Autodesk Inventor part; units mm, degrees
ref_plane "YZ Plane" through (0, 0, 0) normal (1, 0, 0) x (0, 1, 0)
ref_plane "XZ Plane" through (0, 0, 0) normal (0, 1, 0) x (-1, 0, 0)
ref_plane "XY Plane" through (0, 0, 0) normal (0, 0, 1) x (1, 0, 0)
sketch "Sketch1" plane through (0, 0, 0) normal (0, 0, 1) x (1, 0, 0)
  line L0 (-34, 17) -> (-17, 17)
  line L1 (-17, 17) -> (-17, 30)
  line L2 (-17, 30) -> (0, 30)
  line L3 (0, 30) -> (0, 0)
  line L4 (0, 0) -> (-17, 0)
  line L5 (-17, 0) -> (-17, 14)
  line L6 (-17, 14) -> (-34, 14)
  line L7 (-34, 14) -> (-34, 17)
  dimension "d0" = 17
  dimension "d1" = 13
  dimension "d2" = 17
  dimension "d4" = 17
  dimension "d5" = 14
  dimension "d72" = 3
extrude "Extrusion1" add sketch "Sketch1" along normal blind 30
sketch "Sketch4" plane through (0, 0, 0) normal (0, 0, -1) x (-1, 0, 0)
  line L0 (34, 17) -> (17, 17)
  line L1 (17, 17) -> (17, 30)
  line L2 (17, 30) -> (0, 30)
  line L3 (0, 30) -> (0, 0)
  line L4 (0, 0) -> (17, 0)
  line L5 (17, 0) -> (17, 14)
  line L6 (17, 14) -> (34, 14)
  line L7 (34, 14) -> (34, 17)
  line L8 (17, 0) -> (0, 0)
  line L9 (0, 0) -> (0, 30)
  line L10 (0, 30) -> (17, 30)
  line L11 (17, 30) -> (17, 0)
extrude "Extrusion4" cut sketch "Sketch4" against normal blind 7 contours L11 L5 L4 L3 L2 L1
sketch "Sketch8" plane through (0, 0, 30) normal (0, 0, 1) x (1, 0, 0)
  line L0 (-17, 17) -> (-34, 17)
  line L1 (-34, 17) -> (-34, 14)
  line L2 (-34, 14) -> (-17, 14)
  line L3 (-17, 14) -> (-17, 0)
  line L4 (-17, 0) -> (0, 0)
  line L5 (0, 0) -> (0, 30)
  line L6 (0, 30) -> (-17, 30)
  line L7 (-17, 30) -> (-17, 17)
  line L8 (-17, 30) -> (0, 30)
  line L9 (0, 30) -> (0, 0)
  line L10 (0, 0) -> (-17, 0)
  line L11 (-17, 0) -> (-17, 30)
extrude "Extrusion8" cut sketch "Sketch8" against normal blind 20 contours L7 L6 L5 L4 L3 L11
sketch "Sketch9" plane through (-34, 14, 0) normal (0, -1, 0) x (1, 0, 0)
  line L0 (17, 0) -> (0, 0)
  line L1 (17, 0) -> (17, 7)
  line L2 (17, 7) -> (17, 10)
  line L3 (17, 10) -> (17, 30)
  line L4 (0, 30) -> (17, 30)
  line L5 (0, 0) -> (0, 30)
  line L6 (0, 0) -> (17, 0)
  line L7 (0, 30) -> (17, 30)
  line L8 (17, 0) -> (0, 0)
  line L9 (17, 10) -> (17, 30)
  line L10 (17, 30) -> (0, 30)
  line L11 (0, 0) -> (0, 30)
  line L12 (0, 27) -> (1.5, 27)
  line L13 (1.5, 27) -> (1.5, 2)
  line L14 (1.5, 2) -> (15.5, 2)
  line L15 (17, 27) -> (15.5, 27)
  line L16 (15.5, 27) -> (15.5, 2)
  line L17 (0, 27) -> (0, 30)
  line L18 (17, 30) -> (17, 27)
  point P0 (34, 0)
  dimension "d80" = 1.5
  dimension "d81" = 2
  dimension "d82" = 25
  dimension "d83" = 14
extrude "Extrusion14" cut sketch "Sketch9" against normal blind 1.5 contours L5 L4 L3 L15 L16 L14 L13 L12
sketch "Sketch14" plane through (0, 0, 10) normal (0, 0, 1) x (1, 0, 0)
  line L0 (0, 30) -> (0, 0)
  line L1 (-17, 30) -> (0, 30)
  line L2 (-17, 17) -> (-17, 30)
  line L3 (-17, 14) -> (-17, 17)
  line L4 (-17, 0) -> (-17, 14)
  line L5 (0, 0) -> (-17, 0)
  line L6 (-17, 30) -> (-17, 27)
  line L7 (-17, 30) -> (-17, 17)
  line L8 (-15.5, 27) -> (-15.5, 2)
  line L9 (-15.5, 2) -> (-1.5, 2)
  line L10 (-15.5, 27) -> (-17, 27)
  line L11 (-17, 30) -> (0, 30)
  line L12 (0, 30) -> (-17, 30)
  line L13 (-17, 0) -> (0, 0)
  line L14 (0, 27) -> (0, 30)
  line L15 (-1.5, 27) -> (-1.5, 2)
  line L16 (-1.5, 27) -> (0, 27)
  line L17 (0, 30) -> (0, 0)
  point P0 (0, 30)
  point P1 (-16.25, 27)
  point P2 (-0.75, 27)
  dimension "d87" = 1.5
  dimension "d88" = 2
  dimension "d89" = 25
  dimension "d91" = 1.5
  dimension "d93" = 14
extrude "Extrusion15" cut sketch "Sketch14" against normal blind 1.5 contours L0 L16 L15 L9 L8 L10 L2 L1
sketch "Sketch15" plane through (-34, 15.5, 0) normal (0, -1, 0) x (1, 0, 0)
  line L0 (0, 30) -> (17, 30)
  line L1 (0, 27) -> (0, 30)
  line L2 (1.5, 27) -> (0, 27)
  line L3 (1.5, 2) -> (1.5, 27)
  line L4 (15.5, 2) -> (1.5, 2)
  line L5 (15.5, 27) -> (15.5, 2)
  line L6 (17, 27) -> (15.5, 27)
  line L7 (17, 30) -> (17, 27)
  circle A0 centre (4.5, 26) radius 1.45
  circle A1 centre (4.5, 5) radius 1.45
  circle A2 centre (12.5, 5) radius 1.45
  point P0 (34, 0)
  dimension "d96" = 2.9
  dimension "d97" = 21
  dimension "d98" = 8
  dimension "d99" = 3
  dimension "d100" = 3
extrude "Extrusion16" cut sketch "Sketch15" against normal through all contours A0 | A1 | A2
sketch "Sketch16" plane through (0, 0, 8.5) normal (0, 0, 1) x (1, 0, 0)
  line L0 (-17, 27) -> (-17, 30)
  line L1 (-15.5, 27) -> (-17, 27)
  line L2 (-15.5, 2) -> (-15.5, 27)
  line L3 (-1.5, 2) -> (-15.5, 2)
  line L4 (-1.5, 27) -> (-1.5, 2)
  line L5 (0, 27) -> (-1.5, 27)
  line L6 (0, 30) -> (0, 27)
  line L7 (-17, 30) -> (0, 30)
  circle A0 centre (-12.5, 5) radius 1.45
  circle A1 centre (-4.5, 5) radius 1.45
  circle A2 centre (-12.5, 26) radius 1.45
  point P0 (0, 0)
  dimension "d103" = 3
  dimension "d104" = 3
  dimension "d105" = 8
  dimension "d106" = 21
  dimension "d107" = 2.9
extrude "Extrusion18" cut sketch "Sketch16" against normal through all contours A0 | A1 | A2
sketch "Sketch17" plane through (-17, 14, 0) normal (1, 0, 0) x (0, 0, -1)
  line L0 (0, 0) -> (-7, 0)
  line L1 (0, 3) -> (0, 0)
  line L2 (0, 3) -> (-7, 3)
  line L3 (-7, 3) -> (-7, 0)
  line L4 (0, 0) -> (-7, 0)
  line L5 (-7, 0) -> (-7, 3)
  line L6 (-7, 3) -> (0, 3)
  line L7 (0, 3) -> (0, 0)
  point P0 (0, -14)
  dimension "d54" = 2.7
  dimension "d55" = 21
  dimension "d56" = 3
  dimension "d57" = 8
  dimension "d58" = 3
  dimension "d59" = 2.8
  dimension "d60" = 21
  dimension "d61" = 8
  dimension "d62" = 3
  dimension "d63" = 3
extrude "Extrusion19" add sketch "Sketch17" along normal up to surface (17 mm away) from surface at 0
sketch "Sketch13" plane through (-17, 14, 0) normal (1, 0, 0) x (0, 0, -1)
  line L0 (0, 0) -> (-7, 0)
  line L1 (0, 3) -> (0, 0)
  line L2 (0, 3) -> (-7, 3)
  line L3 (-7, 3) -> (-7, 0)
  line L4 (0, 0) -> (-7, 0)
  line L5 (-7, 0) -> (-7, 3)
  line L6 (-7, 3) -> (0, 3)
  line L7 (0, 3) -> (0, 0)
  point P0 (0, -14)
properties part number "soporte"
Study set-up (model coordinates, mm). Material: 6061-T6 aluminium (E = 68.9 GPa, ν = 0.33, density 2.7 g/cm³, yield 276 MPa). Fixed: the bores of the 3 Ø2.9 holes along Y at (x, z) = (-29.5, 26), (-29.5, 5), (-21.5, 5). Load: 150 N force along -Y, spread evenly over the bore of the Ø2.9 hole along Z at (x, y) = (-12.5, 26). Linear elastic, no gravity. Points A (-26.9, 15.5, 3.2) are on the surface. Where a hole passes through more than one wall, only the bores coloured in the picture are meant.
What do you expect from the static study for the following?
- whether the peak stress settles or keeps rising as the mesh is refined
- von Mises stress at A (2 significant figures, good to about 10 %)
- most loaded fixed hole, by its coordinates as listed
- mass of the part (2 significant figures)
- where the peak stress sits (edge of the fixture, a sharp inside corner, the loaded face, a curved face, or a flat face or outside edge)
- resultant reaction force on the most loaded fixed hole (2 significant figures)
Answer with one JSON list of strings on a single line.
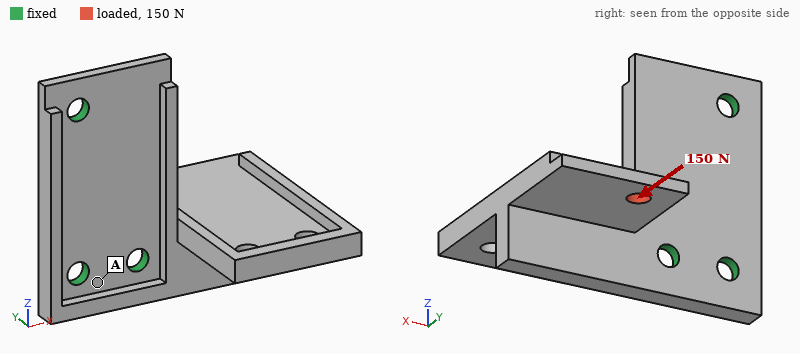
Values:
["keeps rising", "17 MPa", "(-21.5, 5)", "5.8 g", "edge of the fixture", "220 N"]
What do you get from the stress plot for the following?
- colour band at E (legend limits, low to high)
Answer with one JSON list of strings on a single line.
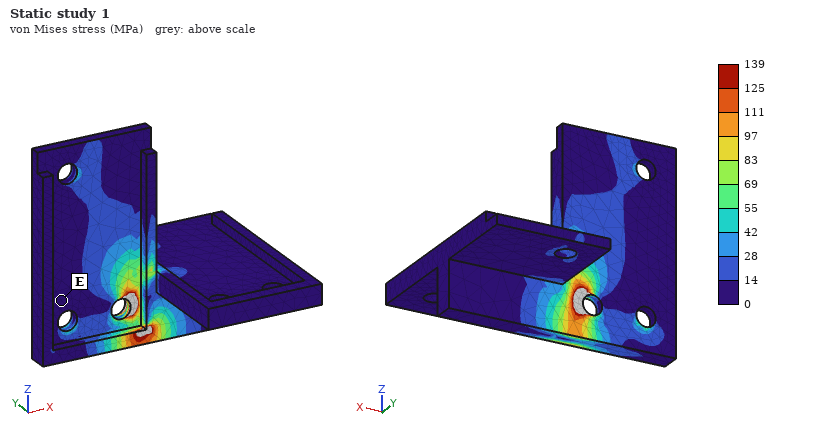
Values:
["0 to 14 MPa"]
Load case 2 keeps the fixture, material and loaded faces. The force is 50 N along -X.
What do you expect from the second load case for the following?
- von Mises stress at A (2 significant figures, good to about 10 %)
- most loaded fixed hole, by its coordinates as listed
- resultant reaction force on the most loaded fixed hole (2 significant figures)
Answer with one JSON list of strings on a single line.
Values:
["7.7 MPa", "(-21.5, 5)", "80 N"]
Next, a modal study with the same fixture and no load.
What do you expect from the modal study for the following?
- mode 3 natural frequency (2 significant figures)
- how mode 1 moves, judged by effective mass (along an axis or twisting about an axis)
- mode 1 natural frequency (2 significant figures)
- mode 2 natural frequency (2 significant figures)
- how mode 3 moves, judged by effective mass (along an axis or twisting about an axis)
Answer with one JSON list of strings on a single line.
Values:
["6800 Hz", "along Y", "2000 Hz", "3900 Hz", "along Z"]
